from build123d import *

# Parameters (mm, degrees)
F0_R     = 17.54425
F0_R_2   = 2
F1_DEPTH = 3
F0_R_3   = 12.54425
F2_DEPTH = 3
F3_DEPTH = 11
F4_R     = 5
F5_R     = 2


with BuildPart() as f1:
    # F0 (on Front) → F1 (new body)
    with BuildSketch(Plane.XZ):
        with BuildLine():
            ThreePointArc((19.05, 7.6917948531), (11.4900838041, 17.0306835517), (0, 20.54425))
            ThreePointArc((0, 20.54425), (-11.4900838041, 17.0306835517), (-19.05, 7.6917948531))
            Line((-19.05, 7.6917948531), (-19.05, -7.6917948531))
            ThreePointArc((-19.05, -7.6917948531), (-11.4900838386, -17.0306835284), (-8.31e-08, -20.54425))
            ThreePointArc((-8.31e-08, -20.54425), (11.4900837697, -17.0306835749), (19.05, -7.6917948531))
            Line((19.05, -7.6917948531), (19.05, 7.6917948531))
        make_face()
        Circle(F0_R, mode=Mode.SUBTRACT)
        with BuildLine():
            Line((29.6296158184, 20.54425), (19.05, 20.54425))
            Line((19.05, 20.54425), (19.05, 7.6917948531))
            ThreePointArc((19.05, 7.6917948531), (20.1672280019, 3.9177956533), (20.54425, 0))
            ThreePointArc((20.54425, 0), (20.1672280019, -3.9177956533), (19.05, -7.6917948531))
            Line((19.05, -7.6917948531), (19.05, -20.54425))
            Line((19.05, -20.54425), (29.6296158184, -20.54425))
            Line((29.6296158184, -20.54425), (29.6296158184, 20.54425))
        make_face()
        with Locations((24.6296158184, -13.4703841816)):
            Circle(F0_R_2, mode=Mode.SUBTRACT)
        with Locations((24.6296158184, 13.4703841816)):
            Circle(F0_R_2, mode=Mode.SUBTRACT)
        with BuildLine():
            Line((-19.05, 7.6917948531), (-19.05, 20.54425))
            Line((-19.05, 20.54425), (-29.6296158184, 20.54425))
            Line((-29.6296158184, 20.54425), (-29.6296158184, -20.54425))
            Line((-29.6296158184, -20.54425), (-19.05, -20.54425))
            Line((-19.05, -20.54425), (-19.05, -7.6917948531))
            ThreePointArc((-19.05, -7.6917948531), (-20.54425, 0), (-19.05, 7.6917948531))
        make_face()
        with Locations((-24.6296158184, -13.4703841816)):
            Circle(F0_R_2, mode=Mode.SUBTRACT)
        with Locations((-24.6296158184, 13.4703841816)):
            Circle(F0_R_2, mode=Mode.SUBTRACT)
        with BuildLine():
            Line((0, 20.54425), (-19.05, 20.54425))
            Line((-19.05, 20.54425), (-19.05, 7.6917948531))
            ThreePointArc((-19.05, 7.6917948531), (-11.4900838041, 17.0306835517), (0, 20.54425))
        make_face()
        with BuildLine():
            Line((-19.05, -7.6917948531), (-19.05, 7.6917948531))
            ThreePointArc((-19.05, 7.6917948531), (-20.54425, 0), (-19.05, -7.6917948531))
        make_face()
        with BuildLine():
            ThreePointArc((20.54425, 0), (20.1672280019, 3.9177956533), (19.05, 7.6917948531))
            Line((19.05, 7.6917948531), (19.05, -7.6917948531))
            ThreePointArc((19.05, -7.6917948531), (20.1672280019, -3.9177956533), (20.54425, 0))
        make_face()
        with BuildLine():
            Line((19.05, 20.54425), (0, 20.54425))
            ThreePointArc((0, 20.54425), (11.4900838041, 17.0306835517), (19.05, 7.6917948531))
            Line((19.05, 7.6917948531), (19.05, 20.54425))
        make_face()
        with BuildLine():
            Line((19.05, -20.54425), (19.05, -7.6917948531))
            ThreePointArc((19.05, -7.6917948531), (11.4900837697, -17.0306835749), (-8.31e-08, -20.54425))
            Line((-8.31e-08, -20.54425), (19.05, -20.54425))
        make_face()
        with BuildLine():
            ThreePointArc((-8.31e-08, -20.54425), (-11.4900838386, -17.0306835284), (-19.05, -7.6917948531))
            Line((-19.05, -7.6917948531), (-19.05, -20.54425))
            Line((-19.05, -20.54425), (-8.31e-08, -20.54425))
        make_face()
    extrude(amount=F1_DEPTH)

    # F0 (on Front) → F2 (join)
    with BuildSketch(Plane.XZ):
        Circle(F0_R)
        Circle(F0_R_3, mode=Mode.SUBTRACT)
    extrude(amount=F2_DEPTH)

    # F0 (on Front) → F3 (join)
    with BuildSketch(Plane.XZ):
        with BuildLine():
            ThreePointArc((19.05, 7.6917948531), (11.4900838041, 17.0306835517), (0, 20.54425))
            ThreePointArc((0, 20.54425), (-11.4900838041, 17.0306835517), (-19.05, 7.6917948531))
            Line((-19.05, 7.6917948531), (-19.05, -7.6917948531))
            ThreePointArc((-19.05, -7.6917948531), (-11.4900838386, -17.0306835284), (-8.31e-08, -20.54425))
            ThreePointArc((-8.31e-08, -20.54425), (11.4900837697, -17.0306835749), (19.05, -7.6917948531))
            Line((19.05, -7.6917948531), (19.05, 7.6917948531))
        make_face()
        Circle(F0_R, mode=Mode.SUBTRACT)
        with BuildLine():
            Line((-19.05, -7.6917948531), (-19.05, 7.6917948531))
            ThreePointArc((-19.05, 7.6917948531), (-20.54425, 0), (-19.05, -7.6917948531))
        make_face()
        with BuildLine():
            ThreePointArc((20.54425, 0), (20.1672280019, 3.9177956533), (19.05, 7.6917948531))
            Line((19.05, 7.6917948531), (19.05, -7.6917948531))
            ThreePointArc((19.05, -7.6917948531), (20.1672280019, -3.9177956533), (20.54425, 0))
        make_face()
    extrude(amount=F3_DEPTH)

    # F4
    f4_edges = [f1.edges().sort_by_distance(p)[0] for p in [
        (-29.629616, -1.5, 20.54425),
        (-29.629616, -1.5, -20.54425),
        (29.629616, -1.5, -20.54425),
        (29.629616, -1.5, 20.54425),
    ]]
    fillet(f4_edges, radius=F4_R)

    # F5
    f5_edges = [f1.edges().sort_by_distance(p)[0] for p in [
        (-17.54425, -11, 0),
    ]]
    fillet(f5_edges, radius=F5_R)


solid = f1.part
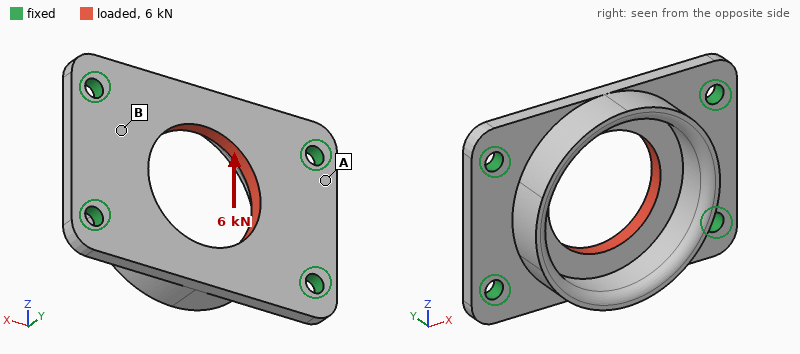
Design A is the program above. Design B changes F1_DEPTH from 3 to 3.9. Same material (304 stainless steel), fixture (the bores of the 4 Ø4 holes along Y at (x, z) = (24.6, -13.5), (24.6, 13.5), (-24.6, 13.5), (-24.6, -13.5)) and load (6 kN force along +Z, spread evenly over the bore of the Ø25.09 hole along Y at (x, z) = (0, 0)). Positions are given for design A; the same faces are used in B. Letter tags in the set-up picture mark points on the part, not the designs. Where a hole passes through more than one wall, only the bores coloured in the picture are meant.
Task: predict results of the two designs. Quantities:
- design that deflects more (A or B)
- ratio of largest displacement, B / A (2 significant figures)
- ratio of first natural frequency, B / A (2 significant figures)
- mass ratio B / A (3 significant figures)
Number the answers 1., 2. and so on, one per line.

1. A
2. 0.91
3. 1.2
4. 1.11
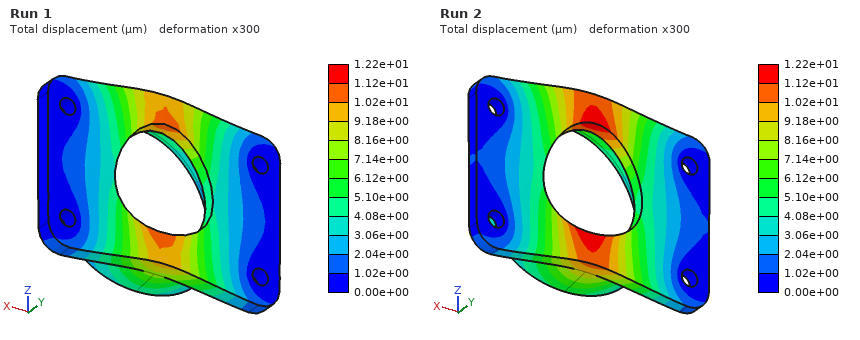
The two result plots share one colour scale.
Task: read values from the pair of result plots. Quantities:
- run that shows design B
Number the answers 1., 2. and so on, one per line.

1. Run 1
